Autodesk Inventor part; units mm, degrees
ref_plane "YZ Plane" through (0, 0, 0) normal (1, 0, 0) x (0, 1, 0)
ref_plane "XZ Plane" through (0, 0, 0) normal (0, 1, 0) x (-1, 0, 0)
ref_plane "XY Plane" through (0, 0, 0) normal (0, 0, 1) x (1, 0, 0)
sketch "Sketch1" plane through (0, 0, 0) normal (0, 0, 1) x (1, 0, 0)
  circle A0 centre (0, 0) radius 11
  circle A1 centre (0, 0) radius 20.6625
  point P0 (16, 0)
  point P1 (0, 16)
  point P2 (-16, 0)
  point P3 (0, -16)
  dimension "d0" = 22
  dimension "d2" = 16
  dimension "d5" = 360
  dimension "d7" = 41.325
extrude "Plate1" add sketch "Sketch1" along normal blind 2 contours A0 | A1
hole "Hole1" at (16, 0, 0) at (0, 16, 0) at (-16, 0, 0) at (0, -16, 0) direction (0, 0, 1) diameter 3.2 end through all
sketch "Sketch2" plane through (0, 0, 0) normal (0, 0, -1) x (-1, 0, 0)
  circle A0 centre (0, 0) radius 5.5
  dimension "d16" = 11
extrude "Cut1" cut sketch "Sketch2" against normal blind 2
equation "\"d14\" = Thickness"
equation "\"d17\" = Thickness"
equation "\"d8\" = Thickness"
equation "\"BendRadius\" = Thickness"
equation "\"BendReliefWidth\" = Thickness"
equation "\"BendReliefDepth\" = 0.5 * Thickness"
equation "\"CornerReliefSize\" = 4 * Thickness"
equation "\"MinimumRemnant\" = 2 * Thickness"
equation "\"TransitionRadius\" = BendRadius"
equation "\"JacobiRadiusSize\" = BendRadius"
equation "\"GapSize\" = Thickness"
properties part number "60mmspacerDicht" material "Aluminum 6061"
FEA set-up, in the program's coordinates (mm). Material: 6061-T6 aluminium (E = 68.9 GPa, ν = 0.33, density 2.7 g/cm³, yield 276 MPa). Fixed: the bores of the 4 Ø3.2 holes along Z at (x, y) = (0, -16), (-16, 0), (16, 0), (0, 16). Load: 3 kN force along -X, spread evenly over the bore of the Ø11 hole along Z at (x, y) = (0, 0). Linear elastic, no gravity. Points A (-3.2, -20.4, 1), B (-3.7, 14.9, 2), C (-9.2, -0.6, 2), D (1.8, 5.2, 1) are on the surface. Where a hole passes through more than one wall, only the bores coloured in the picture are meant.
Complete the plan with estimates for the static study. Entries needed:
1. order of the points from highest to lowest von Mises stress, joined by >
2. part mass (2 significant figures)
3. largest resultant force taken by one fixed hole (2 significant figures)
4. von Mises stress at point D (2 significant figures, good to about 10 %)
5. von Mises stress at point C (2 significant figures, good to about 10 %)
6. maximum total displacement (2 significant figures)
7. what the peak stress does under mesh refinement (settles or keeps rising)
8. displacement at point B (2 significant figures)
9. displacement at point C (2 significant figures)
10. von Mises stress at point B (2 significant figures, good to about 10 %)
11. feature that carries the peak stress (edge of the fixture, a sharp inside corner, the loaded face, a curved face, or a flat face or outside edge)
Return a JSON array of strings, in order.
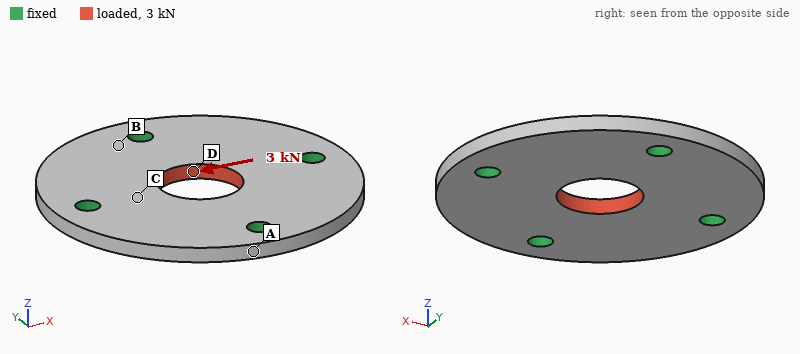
["D > C > B > A", "6.6 g", "940 N", "73 MPa", "56 MPa", "9.5 µm", "keeps rising", "1.6 µm", "5.0 µm", "25 MPa", "edge of the fixture"]
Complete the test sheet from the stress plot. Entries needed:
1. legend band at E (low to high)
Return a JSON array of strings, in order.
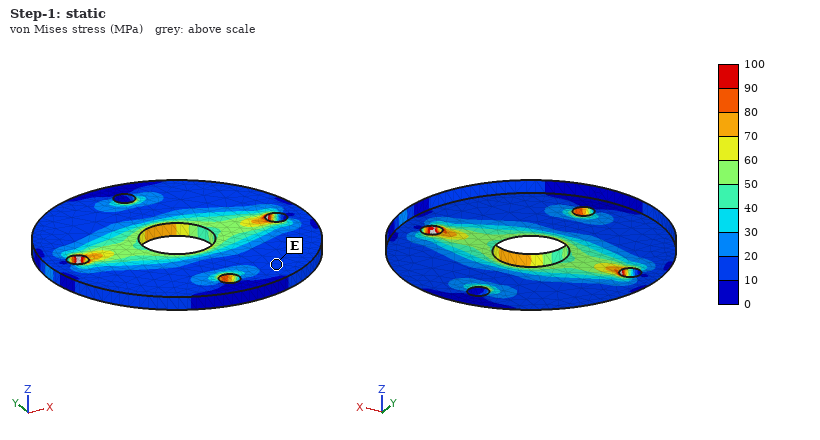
["10 to 20 MPa"]
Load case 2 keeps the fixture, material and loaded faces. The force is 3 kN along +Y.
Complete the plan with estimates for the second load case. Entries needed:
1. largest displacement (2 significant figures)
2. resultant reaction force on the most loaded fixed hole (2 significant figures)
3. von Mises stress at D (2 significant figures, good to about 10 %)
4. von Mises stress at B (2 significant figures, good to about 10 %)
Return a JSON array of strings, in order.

["9.5 µm", "940 N", "47 MPa", "28 MPa"]
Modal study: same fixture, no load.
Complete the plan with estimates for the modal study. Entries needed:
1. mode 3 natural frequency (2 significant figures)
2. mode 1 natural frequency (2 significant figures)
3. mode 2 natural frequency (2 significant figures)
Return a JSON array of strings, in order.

["16 kHz", "15 kHz", "16 kHz"]
